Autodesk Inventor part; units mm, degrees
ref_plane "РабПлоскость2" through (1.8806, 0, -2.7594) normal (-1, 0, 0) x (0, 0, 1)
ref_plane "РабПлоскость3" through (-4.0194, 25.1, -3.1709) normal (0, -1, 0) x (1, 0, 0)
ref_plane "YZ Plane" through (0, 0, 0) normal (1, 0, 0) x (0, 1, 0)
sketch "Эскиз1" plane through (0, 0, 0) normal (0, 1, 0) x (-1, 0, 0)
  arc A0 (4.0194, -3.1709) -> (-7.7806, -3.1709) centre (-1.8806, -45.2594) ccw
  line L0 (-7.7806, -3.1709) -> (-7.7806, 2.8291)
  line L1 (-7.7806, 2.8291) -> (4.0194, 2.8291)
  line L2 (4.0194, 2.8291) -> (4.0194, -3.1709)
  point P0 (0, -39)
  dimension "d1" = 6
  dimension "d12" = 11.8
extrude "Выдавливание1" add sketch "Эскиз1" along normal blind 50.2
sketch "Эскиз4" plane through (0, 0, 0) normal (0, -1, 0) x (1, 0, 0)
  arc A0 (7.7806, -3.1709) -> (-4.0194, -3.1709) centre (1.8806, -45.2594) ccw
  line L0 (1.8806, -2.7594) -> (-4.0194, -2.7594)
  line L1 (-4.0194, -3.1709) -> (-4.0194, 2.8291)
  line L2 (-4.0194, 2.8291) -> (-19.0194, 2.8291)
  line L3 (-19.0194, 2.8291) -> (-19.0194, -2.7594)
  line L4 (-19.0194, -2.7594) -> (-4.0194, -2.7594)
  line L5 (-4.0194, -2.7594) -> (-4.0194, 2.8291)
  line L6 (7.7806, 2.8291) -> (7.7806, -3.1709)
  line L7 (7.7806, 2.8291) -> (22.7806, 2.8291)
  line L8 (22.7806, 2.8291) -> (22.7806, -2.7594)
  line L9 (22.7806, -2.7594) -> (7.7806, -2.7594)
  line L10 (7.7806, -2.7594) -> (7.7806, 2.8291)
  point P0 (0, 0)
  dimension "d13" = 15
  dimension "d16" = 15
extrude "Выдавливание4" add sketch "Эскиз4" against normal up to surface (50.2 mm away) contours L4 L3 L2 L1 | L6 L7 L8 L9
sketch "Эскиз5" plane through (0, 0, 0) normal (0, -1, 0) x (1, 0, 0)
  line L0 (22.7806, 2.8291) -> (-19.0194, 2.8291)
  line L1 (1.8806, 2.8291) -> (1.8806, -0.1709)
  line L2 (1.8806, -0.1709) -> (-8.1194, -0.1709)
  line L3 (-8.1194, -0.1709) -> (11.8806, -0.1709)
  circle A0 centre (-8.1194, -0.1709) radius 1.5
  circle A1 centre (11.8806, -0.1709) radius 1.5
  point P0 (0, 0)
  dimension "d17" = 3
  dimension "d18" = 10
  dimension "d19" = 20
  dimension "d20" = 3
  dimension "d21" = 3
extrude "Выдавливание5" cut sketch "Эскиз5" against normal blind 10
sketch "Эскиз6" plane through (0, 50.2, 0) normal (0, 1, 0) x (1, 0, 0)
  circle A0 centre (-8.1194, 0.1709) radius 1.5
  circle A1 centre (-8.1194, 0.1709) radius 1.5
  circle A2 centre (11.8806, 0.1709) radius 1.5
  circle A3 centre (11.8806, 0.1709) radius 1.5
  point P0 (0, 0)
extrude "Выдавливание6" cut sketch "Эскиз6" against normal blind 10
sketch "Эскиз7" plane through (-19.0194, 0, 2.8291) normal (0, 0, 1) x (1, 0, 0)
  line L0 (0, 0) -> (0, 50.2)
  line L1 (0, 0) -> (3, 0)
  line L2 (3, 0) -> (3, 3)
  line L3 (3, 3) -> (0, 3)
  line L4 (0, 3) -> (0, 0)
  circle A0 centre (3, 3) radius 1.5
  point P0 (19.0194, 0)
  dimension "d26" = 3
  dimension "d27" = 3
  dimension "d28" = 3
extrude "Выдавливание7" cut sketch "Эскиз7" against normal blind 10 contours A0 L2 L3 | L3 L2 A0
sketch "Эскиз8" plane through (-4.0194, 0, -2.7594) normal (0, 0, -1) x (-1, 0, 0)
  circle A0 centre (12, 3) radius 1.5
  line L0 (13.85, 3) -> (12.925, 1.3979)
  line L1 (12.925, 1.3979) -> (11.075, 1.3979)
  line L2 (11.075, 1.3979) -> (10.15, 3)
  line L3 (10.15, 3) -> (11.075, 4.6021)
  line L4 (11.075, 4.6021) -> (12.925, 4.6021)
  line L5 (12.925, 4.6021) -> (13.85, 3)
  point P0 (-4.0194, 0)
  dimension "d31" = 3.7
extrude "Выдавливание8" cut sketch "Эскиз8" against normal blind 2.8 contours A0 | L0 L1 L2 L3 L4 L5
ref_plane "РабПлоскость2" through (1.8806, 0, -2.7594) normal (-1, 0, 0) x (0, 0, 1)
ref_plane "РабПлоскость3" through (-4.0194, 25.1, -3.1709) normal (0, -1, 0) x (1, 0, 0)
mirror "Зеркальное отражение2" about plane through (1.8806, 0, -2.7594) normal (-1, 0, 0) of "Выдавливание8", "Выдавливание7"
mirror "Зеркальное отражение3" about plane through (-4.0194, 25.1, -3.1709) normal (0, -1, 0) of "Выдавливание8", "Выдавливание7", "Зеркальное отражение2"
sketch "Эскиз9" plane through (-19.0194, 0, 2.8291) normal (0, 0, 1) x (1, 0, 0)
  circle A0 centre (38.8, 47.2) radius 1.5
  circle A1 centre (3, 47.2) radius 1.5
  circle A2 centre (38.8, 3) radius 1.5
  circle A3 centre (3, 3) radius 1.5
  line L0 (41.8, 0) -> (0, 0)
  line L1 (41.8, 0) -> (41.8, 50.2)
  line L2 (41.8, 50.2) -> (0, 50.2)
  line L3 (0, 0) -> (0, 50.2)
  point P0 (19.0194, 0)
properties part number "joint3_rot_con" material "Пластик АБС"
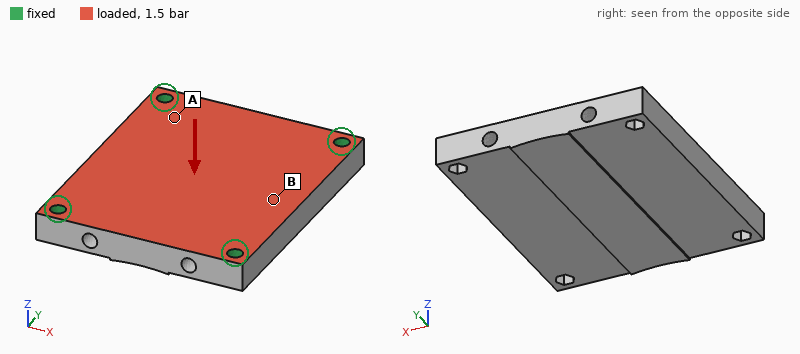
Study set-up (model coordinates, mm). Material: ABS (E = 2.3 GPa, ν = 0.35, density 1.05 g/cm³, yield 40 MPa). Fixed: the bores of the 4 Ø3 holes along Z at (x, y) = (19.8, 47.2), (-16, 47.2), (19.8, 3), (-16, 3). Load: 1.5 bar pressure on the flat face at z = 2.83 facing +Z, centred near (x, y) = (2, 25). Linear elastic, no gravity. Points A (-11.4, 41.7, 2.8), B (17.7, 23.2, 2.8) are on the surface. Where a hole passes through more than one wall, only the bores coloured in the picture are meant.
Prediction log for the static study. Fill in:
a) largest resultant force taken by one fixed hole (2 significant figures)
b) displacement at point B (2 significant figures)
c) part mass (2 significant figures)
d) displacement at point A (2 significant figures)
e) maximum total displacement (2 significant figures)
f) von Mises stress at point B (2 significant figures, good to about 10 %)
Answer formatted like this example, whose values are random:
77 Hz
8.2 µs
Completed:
95 N
0.11 mm
12 g
0.054 mm
0.14 mm
3.3 MPa
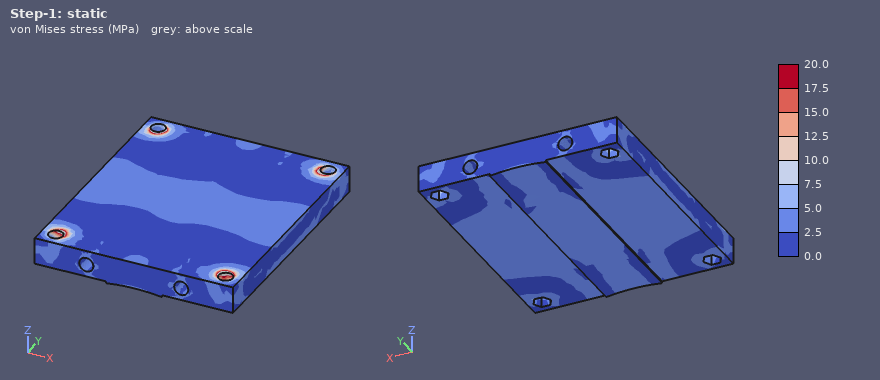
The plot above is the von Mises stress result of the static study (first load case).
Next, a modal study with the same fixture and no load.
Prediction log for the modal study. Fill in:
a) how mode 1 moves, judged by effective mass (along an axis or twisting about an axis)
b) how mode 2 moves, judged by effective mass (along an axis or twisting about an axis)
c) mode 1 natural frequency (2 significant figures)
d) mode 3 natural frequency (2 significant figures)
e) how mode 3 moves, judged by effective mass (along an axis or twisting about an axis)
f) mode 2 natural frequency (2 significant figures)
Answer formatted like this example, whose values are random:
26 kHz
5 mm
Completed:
along Z
twisting about Y
2500 Hz
4800 Hz
twisting about X
4000 Hz
